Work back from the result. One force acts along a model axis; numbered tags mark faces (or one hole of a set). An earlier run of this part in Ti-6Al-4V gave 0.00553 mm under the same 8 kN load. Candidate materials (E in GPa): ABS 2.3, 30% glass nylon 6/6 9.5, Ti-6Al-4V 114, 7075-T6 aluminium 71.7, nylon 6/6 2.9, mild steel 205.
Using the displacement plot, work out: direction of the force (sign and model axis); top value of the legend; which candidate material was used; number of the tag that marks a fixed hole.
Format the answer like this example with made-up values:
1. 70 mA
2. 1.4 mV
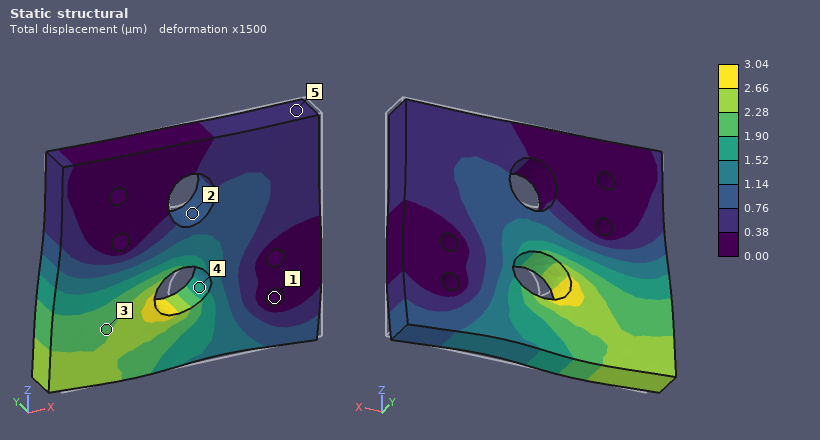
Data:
1. -X
2. 3.04 µm
3. mild steel
4. 1
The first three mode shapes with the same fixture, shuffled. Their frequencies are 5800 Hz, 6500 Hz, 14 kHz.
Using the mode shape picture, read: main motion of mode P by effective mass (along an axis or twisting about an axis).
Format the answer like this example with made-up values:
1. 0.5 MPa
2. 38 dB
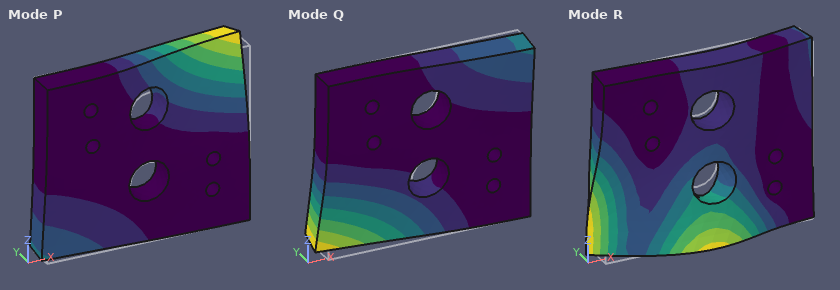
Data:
1. along Y
